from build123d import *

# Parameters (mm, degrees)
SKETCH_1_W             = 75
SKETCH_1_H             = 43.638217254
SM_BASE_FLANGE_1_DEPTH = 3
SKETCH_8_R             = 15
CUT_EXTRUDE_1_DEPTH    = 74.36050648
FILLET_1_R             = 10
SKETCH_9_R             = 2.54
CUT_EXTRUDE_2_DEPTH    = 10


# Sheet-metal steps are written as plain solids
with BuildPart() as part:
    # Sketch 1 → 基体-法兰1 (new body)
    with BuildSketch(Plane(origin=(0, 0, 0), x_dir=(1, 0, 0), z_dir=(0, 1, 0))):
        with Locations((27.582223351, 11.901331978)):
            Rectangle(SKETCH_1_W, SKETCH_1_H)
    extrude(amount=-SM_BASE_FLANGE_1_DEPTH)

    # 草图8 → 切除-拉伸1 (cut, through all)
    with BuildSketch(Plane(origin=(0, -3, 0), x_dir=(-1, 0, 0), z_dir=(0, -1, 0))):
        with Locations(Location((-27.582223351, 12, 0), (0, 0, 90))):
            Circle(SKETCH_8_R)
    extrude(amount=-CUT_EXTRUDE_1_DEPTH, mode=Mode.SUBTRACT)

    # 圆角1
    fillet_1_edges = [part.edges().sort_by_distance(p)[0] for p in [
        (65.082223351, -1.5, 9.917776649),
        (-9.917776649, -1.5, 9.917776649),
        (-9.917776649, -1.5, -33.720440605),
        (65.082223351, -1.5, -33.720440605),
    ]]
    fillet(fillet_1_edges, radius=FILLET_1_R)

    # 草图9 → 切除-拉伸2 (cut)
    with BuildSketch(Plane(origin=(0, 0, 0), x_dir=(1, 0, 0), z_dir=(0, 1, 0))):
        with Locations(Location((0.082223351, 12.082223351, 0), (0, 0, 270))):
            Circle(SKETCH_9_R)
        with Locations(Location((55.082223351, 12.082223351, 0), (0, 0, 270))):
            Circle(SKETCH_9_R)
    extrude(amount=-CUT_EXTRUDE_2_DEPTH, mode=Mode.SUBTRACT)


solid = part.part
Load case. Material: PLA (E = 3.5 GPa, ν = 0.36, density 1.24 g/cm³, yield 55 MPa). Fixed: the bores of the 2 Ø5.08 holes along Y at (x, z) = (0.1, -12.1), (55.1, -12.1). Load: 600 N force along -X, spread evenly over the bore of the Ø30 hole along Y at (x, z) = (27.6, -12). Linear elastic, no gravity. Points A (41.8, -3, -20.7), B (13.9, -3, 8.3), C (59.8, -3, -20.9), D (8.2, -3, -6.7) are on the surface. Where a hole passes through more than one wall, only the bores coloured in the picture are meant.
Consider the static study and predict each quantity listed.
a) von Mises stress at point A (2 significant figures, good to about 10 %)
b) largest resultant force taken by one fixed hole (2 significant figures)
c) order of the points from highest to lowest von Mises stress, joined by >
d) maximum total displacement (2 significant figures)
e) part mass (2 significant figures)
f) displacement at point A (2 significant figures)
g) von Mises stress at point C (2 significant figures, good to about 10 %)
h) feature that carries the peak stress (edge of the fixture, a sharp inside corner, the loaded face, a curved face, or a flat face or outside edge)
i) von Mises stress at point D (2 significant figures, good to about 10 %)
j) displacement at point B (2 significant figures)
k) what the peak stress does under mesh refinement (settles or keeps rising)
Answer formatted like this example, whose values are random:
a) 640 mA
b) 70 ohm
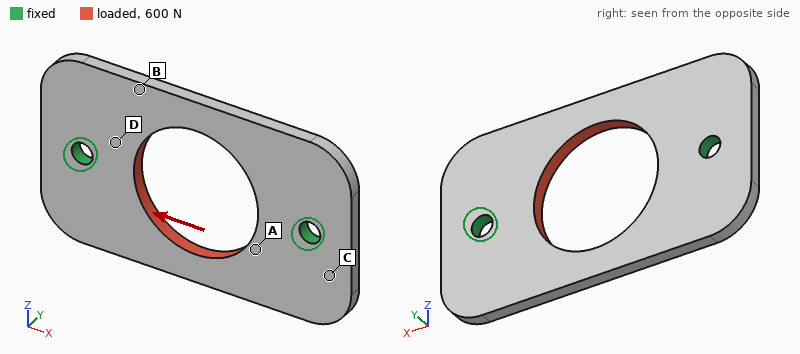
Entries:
a) 4.0 MPa
b) 300 N
c) D > A > C > B
d) 49 µm
e) 9.1 g
f) 29 µm
g) 2.3 MPa
h) edge of the fixture
i) 5.1 MPa
j) 40 µm
k) keeps rising
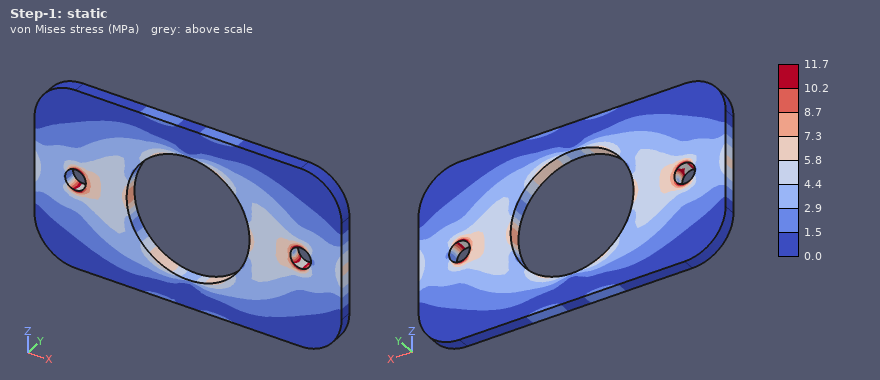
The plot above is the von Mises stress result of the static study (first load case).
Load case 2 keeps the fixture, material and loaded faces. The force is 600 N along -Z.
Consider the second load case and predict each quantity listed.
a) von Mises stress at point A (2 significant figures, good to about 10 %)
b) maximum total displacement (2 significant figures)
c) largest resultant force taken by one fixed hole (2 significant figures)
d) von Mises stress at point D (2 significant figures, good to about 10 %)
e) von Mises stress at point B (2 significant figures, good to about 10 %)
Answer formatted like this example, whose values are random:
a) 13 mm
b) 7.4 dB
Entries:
a) 6.4 MPa
b) 90 µm
c) 300 N
d) 6.3 MPa
e) 3.1 MPa
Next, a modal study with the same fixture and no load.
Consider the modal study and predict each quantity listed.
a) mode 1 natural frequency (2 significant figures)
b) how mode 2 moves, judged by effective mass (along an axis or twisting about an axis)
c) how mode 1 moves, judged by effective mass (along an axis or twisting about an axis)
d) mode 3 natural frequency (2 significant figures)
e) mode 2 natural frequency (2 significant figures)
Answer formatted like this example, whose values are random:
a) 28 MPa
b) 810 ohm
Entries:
a) 1200 Hz
b) along Y
c) twisting about X
d) 2000 Hz
e) 1300 Hz
